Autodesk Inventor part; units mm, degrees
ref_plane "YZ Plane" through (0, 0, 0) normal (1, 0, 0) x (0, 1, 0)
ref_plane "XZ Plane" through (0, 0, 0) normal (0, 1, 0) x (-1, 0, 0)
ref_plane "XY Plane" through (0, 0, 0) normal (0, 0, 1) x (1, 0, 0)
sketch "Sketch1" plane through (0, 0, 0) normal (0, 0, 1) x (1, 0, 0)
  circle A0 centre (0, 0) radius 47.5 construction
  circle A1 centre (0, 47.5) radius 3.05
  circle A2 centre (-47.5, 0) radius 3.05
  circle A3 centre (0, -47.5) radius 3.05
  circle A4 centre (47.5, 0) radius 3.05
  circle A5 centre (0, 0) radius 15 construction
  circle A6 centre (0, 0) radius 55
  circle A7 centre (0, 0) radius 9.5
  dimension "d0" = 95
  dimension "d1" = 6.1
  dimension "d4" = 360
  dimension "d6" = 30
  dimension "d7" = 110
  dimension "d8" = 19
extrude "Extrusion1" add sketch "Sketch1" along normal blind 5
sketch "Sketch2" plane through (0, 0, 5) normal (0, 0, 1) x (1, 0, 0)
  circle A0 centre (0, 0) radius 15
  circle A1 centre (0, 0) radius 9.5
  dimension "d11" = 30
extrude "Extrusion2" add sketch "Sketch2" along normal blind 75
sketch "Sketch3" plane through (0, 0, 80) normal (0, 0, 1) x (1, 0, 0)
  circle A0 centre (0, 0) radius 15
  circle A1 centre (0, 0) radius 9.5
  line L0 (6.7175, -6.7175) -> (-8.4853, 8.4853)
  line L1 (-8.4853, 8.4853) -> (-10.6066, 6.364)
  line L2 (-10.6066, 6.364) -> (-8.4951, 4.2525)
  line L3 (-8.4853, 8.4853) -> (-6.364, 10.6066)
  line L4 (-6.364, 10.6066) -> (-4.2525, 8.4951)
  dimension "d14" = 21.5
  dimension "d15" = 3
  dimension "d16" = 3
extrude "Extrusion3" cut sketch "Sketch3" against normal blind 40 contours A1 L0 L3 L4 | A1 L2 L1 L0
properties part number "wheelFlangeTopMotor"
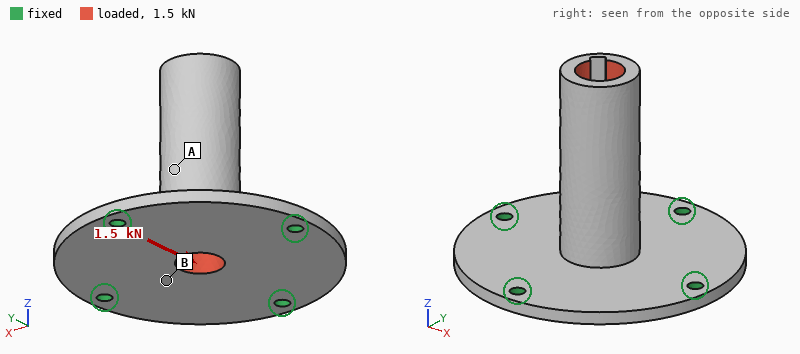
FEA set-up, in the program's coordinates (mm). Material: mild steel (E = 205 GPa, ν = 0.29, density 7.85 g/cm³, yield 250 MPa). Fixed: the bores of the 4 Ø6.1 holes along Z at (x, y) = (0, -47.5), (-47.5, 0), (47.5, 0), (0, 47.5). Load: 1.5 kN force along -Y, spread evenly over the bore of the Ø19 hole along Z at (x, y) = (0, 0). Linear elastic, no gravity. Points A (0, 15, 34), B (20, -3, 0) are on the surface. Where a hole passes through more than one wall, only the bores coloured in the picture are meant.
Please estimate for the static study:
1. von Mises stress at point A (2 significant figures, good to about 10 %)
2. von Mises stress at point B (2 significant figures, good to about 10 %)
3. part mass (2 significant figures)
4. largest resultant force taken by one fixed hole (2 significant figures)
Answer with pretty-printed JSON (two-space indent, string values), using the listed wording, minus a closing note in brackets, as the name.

{
  "von Mises stress at point A": "8.5 MPa",
  "von Mises stress at point B": "31 MPa",
  "part mass": "600 g",
  "largest resultant force taken by one fixed hole": "860 N"
}
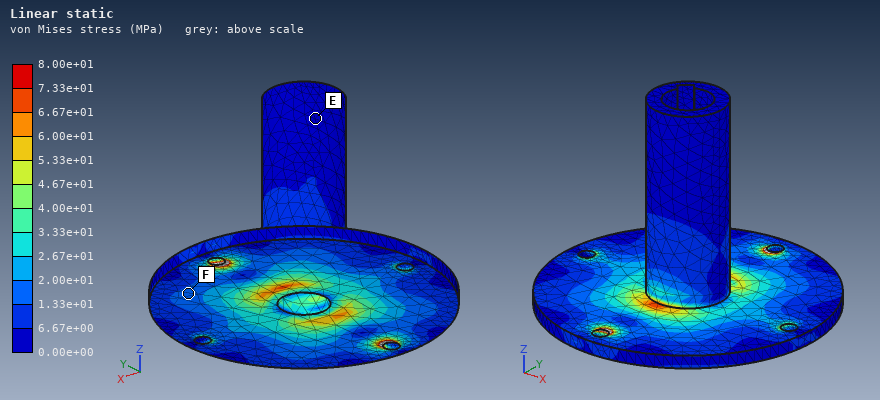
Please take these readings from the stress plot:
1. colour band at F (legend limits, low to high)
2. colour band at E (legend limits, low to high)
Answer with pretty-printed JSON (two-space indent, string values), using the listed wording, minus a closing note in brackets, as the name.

{
  "colour band at F": "1.33e+01 to 2.00e+01 MPa",
  "colour band at E": "0.00e+00 to 6.67e+00 MPa"
}
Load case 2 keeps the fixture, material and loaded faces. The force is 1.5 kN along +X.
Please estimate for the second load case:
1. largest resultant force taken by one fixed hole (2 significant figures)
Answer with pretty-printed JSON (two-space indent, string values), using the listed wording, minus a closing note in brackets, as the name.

{
  "largest resultant force taken by one fixed hole": "860 N"
}
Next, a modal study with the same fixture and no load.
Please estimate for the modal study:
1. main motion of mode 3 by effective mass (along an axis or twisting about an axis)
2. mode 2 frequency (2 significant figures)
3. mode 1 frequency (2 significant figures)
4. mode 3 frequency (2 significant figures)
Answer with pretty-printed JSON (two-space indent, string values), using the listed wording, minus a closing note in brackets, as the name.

{
  "main motion of mode 3 by effective mass": "along Z",
  "mode 2 frequency": "1400 Hz",
  "mode 1 frequency": "1400 Hz",
  "mode 3 frequency": "2400 Hz"
}
